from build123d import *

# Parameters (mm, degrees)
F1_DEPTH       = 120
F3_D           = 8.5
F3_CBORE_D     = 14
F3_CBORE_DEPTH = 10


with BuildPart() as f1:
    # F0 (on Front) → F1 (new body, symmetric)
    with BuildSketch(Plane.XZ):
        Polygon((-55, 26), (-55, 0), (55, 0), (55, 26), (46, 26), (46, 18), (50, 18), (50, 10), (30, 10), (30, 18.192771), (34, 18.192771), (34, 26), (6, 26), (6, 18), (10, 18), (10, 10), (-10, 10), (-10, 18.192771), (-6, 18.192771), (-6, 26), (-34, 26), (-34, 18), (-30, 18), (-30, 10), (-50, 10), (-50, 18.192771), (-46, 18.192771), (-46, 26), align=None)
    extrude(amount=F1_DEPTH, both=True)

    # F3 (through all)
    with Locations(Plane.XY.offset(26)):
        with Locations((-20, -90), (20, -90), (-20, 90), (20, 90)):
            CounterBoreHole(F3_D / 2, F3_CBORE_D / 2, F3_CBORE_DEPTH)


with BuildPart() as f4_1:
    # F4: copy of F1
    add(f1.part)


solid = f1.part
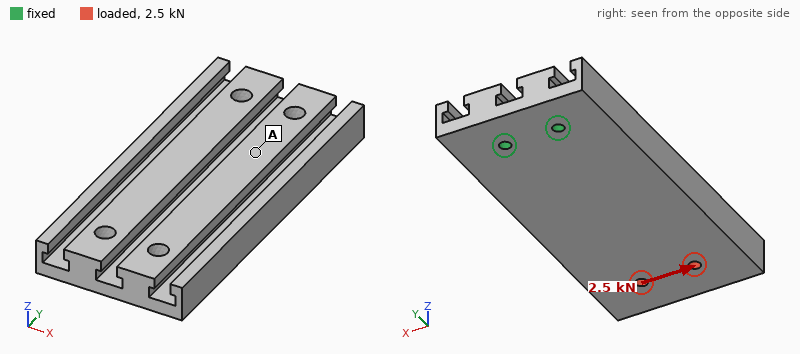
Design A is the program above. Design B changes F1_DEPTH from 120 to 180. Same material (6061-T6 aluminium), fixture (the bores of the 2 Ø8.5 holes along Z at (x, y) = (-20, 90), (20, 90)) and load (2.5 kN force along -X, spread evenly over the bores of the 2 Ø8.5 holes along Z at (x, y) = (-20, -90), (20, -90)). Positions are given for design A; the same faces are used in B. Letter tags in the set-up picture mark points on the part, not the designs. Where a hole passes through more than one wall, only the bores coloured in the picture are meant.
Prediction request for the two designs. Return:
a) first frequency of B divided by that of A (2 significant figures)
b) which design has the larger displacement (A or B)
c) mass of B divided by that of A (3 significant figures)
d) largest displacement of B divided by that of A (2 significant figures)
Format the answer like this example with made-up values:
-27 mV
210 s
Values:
0.63
B
1.51
1.2
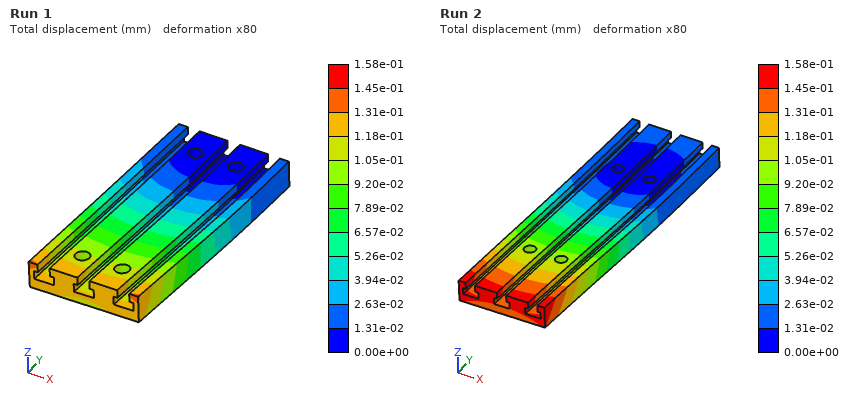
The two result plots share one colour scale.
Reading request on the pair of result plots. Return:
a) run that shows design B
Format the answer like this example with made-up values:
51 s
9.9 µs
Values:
Run 2
